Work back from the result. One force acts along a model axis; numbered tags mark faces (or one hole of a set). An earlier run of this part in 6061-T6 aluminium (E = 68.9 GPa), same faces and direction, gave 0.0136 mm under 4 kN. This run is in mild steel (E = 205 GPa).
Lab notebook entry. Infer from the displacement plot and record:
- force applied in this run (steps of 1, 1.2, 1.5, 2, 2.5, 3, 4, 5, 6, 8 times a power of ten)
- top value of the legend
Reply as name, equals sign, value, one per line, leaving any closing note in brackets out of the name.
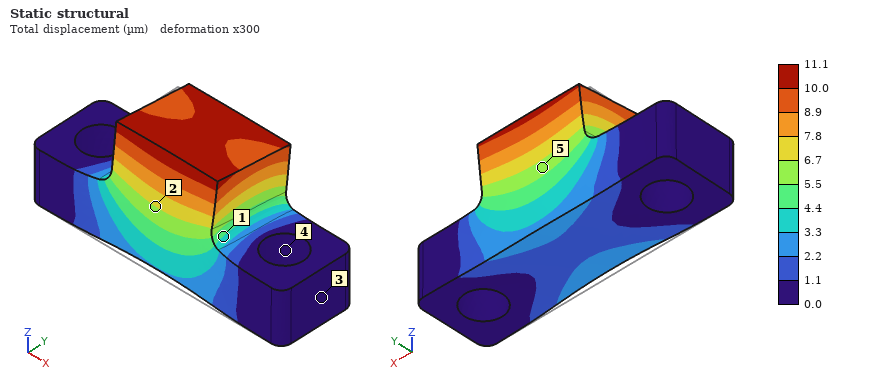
force applied in this run = 10 kN
top value of the legend = 11.1 µm
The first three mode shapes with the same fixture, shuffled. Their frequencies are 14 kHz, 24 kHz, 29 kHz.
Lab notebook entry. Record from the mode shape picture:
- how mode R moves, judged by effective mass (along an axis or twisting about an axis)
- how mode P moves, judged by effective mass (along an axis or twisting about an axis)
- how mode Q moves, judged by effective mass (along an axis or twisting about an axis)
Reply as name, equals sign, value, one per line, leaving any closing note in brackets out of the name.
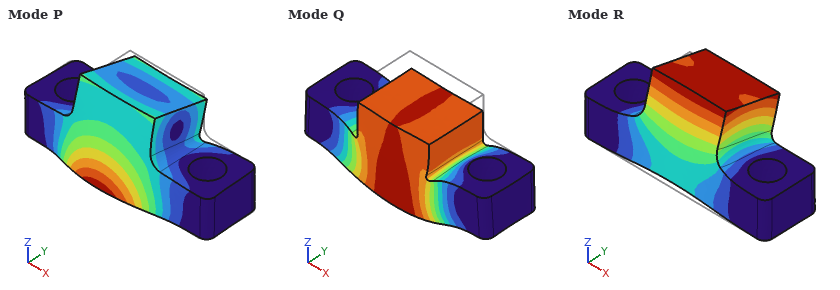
how mode R moves, judged by effective mass = along Y
how mode P moves, judged by effective mass = along Y
how mode Q moves, judged by effective mass = along Z
